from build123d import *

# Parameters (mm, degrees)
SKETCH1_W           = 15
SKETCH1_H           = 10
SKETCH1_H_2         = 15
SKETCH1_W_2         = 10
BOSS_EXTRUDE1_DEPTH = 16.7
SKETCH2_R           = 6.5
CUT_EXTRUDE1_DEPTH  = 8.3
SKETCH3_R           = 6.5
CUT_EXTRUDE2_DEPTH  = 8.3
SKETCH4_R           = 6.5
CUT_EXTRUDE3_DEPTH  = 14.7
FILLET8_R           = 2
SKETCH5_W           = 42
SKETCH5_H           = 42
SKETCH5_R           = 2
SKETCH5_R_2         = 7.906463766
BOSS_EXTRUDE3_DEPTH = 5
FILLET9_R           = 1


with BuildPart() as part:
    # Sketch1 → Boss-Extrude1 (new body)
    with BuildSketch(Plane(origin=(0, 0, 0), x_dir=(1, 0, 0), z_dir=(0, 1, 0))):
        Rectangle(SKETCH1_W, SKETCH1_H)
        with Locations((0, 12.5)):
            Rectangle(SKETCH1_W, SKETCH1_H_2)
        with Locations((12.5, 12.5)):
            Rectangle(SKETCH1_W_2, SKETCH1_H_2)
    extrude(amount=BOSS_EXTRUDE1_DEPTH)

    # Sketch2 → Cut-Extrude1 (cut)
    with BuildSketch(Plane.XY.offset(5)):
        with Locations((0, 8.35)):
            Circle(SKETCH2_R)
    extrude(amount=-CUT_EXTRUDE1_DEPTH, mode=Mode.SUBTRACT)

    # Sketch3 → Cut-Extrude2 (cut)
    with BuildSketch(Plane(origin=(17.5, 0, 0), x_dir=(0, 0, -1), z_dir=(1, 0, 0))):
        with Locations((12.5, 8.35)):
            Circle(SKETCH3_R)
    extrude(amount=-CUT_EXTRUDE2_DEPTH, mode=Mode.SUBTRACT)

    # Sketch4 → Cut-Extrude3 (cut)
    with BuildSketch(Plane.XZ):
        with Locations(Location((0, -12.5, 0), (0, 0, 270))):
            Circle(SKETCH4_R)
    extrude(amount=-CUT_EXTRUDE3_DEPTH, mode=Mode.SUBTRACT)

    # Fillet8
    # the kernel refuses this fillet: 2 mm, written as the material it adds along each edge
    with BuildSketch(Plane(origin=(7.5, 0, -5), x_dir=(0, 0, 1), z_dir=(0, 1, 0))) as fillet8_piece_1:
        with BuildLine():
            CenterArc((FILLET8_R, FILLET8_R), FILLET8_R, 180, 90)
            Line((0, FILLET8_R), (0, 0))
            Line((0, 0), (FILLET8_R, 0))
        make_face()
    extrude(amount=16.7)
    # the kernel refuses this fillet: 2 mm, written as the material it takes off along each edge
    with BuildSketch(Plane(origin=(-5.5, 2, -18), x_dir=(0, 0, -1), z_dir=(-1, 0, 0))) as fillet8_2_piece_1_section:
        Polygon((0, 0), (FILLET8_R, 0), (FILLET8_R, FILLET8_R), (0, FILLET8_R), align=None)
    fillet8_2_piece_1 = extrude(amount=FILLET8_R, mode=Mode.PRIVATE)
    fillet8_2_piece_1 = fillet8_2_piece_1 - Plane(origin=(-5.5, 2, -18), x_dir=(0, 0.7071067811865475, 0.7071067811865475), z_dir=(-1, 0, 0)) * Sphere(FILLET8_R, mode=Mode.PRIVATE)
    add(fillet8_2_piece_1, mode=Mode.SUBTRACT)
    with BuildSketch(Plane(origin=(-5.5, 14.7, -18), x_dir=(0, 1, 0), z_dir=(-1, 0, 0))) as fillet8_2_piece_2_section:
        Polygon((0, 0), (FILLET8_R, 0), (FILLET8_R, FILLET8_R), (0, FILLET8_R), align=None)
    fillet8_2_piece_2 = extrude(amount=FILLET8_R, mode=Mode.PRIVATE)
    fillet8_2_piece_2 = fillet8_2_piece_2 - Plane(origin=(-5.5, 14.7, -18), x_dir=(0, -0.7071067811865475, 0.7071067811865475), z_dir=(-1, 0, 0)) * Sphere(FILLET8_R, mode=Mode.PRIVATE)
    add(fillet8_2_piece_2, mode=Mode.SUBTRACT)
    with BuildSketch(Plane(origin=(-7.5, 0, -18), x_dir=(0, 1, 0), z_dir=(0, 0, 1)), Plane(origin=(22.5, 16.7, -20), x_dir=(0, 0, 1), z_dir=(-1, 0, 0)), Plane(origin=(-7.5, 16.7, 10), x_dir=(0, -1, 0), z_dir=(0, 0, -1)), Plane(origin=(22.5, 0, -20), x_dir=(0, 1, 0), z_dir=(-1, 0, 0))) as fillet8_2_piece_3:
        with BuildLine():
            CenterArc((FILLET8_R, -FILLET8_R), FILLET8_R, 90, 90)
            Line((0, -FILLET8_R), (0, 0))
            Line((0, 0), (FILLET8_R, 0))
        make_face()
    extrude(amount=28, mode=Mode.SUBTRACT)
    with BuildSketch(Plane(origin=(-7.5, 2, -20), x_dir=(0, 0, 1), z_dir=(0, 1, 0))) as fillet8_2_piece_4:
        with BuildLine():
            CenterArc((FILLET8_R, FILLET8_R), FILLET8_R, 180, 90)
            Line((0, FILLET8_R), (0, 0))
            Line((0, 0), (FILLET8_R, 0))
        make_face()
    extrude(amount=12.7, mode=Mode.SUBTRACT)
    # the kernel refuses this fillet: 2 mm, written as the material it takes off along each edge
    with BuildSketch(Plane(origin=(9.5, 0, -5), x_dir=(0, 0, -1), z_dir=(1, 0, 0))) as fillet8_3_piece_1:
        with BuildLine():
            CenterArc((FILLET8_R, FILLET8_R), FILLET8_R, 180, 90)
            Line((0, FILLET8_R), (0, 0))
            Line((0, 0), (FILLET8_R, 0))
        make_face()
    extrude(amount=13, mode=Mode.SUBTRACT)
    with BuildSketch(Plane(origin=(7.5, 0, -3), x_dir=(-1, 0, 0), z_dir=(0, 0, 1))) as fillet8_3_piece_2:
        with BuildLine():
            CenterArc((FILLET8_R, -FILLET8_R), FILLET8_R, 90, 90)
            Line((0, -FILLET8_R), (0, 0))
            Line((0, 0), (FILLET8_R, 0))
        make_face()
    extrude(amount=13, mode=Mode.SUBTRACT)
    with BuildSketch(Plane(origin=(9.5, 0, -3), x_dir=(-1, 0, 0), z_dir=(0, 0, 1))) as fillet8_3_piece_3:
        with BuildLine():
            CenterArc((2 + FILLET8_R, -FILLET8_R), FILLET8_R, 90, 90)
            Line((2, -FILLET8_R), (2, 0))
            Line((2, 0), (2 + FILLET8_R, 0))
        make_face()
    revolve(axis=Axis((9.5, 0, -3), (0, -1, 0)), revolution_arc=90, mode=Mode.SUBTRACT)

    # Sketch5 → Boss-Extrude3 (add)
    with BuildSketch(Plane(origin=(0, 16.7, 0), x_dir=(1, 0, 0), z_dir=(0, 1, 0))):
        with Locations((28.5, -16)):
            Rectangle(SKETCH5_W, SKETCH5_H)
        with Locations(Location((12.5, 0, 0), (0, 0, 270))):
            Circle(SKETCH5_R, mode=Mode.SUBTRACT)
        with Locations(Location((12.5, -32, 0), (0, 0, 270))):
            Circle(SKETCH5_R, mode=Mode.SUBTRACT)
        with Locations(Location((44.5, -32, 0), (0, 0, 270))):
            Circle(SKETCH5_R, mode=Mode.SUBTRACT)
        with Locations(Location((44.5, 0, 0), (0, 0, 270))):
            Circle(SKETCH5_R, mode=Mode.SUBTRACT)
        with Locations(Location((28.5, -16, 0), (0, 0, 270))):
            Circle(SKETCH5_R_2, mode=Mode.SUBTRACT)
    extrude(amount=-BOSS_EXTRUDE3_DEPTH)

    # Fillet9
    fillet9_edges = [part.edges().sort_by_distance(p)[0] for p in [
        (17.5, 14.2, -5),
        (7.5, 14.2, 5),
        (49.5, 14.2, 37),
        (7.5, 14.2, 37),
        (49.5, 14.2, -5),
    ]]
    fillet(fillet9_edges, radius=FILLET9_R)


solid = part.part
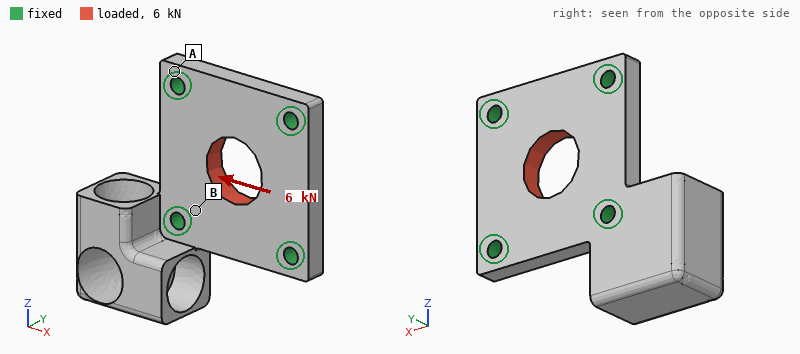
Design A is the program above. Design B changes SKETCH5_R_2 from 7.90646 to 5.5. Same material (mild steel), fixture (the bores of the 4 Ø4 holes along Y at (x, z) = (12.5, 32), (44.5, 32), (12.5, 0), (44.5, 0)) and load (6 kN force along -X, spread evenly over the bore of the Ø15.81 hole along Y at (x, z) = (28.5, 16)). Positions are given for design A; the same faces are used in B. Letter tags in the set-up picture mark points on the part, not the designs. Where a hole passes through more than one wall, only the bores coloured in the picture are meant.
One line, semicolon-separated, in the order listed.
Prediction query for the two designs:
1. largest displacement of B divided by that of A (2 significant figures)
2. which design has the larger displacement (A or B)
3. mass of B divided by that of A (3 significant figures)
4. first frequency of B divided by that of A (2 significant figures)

1.1; B; 1.04; 1.0
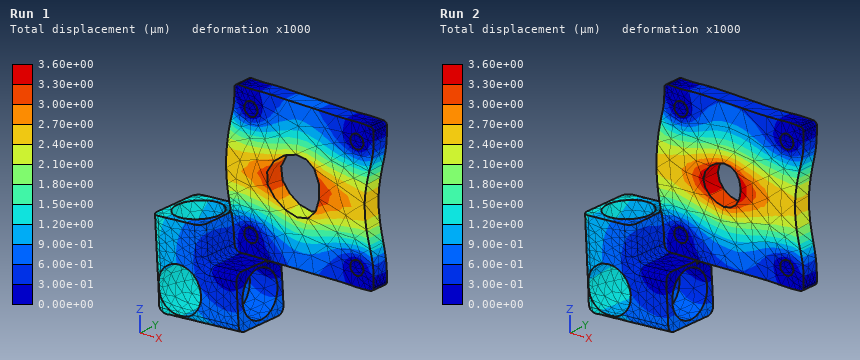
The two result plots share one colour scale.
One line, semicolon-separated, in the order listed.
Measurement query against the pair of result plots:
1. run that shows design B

Run 2
